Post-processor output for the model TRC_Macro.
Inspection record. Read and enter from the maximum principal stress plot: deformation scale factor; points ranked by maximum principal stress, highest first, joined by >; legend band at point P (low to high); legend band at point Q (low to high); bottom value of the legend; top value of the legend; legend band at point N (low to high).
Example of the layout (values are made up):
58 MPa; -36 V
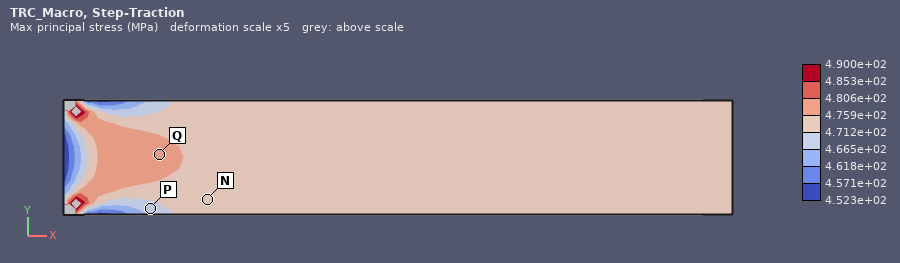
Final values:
5; Q > N > P; 4.665e+02 to 4.712e+02 MPa; 4.759e+02 to 4.806e+02 MPa; 4.523e+02 MPa; 4.900e+02 MPa; 4.712e+02 to 4.759e+02 MPa
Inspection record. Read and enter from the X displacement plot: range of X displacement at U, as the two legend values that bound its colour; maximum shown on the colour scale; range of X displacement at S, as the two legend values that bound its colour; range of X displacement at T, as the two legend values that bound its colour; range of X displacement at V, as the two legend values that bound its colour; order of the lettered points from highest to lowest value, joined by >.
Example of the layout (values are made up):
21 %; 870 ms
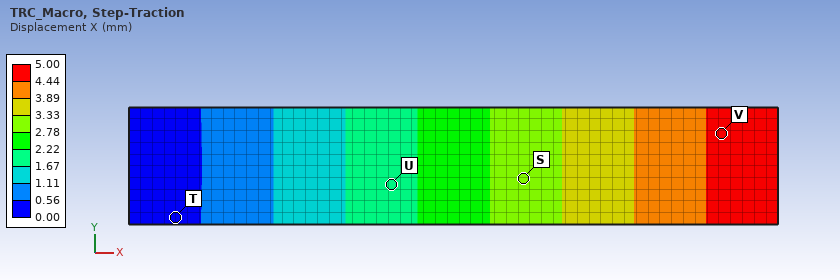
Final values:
1.67 to 2.22 mm; 5.00 mm; 2.78 to 3.33 mm; 0.00 to 0.56 mm; 4.44 to 5.00 mm; V > S > U > T
